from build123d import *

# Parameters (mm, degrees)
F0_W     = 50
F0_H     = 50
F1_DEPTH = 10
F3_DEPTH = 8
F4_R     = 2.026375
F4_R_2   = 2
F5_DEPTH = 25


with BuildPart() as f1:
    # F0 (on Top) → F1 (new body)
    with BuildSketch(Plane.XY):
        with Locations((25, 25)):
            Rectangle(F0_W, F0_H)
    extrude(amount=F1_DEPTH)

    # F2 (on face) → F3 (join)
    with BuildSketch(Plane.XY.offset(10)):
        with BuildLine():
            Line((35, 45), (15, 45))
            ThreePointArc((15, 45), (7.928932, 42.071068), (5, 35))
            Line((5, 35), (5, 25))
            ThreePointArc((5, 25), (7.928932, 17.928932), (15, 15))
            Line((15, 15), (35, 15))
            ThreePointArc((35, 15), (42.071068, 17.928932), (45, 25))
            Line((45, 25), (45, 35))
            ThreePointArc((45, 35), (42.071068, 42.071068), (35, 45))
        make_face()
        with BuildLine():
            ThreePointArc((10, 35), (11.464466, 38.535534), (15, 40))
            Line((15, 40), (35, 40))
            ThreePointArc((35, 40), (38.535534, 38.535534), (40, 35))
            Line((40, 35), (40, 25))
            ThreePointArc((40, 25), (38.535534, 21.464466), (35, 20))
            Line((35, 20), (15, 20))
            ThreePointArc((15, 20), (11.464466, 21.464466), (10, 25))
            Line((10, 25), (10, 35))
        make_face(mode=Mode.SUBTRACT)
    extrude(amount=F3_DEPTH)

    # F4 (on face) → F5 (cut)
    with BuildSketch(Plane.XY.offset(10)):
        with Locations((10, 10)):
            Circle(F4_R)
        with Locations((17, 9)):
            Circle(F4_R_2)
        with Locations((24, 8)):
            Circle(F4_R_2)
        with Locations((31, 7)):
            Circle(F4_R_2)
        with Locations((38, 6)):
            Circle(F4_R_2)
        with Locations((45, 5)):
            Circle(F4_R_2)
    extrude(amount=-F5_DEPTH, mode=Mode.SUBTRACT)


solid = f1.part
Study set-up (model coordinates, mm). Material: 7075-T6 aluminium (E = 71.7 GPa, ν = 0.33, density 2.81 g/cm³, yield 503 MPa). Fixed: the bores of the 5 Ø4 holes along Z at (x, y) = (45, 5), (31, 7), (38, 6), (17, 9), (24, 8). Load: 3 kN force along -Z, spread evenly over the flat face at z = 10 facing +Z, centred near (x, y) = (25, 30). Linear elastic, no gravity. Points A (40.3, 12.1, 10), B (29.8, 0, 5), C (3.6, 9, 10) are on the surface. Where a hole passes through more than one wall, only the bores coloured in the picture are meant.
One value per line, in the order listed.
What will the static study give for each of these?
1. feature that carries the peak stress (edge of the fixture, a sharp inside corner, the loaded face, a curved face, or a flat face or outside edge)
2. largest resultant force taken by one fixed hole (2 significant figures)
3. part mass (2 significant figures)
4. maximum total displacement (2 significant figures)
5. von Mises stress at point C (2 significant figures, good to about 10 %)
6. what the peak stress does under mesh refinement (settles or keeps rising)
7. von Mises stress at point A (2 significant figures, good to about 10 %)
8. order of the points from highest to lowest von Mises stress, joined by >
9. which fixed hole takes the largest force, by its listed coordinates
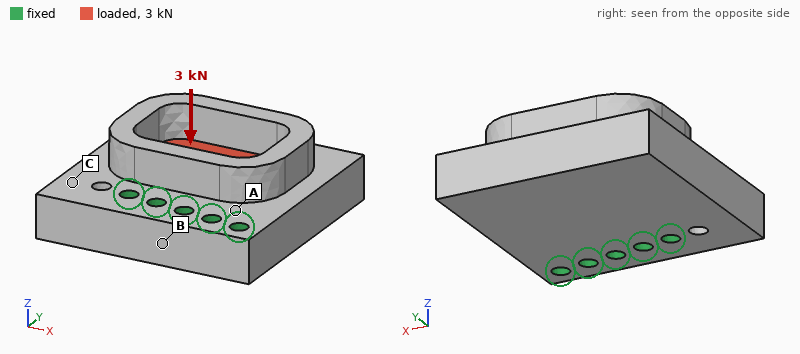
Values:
edge of the fixture
1.3 kN
80 g
92 µm
21 MPa
keeps rising
55 MPa
A > C > B
(17, 9)
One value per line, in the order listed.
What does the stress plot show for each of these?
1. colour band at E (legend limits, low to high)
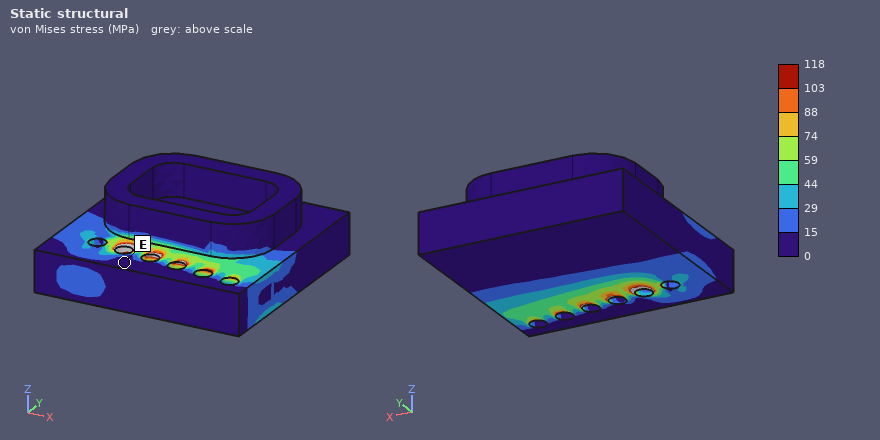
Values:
0 to 15 MPa
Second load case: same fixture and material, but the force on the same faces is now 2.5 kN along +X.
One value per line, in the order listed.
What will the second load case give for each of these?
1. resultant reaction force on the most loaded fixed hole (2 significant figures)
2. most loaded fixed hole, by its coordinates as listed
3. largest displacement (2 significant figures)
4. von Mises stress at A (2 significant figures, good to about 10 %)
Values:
2.1 kN
(17, 9)
18 µm
16 MPa
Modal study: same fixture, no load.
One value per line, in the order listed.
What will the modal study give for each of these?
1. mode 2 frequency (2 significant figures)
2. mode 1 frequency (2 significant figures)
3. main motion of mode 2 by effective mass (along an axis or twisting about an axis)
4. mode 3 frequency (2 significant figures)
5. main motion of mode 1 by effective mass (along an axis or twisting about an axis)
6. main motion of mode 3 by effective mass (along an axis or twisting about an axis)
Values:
7700 Hz
4100 Hz
twisting about Y
9500 Hz
along Z
along X
